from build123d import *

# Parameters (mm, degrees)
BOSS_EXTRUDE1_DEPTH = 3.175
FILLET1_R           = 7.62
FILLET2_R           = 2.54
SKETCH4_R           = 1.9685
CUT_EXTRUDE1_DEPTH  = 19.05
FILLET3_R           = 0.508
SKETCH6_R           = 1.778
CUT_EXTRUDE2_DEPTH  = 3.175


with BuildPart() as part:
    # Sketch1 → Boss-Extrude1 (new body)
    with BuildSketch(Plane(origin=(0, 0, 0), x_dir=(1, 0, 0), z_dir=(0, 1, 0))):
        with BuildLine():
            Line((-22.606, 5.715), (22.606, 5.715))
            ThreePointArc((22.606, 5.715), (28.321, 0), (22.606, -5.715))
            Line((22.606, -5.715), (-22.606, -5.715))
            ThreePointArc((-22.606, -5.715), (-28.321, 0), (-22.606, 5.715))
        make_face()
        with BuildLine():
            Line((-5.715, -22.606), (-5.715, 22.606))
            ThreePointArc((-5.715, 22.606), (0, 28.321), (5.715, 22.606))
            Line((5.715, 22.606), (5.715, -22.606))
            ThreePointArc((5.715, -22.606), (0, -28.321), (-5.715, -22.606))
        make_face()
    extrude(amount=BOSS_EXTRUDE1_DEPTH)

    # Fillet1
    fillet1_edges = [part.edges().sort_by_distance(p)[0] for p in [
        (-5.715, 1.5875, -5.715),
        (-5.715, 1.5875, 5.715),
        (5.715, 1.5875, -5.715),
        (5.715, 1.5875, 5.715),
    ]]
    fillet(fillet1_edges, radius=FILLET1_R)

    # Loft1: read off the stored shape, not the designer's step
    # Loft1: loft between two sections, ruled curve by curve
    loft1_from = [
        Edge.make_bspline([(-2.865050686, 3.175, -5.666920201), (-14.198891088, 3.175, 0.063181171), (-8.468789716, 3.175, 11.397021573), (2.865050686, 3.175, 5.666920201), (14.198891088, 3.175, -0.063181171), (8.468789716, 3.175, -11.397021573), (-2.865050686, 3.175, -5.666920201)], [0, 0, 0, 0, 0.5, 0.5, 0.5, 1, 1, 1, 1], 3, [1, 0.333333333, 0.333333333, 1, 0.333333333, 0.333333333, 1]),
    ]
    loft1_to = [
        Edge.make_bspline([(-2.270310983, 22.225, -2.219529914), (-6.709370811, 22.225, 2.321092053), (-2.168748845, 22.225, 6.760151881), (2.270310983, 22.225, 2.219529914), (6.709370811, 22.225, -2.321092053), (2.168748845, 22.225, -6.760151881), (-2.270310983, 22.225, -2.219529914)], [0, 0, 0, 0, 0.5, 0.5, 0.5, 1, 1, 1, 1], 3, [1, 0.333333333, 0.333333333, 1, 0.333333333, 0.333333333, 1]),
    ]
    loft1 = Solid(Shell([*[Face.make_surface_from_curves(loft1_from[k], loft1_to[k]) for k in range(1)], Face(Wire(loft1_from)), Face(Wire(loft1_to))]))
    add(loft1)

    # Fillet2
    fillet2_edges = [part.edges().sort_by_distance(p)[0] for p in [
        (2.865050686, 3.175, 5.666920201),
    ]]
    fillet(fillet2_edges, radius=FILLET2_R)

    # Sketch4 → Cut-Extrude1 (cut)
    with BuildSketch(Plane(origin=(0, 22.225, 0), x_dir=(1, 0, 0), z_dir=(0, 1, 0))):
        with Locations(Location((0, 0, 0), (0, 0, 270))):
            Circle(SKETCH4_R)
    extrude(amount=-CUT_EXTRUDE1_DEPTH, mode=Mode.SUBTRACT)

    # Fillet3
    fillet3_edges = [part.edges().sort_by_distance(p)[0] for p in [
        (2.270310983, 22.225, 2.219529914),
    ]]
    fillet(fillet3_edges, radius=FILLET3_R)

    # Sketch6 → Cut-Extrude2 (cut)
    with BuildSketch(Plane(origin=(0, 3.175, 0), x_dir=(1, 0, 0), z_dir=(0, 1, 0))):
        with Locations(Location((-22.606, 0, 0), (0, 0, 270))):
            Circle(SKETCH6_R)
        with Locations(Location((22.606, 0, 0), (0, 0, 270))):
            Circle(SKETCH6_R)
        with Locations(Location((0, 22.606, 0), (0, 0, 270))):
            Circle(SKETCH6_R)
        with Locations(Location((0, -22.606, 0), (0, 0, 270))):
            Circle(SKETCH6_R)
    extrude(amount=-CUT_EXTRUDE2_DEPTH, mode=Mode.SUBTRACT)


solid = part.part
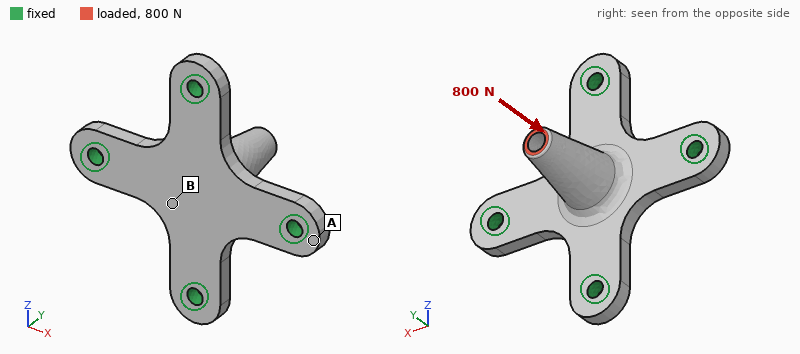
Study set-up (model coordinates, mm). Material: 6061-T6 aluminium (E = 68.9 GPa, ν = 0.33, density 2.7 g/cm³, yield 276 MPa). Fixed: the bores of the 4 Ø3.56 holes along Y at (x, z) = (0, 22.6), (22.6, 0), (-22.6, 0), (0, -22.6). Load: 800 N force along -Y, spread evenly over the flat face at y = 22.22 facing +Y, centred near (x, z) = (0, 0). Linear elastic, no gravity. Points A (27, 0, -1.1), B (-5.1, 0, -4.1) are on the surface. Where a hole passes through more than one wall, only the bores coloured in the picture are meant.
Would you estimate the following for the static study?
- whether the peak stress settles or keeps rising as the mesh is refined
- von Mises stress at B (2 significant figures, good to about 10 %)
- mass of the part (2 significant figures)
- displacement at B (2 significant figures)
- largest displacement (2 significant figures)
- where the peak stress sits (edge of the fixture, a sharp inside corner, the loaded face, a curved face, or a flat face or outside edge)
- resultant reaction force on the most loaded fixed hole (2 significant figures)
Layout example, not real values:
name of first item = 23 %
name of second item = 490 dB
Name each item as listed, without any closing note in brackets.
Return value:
whether the peak stress settles or keeps rising as the mesh is refined = keeps rising
von Mises stress at B = 34 MPa
mass of the part = 13 g
displacement at B = 35 µm
largest displacement = 41 µm
where the peak stress sits = edge of the fixture
resultant reaction force on the most loaded fixed hole = 210 N
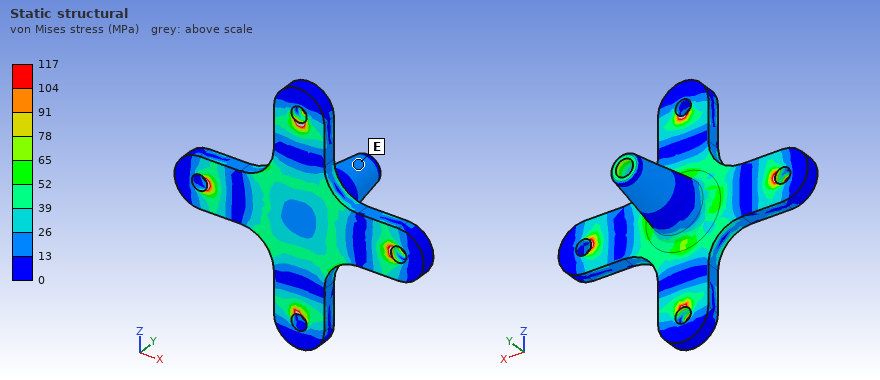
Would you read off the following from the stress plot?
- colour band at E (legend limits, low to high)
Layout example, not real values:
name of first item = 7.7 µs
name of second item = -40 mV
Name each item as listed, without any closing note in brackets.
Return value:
colour band at E = 13 to 26 MPa
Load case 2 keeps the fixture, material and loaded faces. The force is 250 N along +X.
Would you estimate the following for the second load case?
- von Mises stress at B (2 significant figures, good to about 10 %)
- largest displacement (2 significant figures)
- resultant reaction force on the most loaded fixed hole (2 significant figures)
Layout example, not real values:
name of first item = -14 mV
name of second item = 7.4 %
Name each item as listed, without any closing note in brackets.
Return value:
von Mises stress at B = 25 MPa
largest displacement = 58 µm
resultant reaction force on the most loaded fixed hole = 180 N
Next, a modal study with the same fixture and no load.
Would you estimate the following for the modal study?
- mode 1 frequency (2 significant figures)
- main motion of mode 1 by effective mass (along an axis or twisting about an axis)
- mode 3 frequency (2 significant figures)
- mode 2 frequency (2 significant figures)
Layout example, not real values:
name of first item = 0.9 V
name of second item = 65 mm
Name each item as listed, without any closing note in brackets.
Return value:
mode 1 frequency = 9000 Hz
main motion of mode 1 by effective mass = along Y
mode 3 frequency = 12 kHz
mode 2 frequency = 12 kHz
